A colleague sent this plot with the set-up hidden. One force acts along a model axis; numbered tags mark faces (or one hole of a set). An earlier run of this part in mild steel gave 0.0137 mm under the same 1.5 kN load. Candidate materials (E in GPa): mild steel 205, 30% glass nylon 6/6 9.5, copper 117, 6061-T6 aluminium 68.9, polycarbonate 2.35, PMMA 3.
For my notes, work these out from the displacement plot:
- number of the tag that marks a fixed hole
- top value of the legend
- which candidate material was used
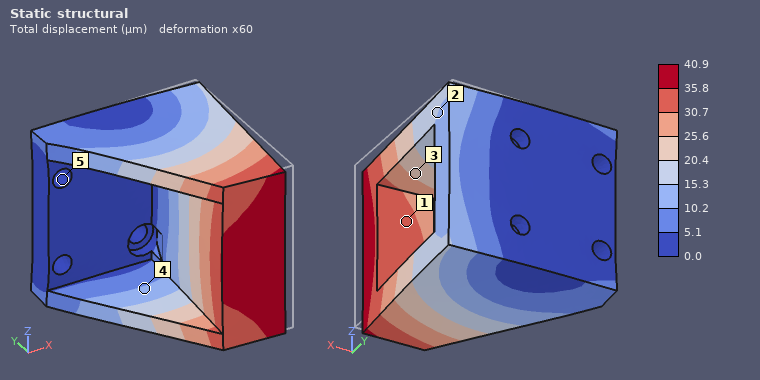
5
40.9 µm
6061-T6 aluminium
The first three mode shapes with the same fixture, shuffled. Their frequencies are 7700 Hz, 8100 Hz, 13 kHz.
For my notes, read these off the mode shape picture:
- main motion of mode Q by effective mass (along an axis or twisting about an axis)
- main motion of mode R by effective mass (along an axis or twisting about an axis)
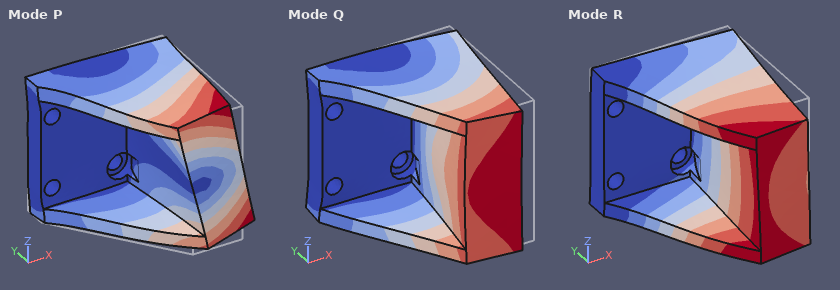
along X
along Z
